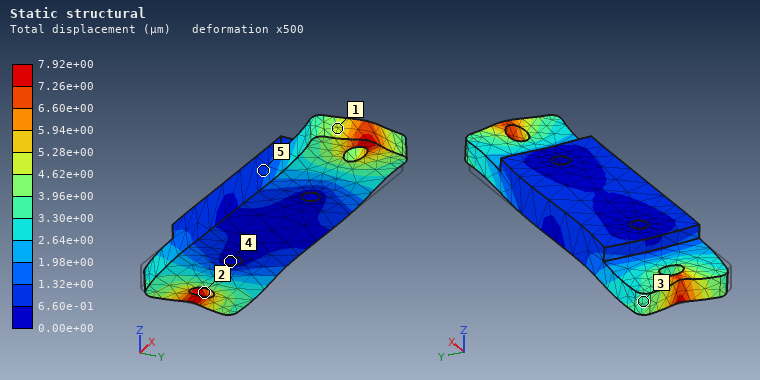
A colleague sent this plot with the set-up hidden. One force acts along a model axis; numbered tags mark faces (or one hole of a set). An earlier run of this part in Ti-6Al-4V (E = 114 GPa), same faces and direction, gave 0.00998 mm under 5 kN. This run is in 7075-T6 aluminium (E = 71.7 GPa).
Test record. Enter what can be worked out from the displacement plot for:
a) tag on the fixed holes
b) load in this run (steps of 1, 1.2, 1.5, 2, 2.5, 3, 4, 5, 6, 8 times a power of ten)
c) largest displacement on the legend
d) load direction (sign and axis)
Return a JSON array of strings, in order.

["4", "2.5 kN", "7.92e+00 µm", "+X"]
